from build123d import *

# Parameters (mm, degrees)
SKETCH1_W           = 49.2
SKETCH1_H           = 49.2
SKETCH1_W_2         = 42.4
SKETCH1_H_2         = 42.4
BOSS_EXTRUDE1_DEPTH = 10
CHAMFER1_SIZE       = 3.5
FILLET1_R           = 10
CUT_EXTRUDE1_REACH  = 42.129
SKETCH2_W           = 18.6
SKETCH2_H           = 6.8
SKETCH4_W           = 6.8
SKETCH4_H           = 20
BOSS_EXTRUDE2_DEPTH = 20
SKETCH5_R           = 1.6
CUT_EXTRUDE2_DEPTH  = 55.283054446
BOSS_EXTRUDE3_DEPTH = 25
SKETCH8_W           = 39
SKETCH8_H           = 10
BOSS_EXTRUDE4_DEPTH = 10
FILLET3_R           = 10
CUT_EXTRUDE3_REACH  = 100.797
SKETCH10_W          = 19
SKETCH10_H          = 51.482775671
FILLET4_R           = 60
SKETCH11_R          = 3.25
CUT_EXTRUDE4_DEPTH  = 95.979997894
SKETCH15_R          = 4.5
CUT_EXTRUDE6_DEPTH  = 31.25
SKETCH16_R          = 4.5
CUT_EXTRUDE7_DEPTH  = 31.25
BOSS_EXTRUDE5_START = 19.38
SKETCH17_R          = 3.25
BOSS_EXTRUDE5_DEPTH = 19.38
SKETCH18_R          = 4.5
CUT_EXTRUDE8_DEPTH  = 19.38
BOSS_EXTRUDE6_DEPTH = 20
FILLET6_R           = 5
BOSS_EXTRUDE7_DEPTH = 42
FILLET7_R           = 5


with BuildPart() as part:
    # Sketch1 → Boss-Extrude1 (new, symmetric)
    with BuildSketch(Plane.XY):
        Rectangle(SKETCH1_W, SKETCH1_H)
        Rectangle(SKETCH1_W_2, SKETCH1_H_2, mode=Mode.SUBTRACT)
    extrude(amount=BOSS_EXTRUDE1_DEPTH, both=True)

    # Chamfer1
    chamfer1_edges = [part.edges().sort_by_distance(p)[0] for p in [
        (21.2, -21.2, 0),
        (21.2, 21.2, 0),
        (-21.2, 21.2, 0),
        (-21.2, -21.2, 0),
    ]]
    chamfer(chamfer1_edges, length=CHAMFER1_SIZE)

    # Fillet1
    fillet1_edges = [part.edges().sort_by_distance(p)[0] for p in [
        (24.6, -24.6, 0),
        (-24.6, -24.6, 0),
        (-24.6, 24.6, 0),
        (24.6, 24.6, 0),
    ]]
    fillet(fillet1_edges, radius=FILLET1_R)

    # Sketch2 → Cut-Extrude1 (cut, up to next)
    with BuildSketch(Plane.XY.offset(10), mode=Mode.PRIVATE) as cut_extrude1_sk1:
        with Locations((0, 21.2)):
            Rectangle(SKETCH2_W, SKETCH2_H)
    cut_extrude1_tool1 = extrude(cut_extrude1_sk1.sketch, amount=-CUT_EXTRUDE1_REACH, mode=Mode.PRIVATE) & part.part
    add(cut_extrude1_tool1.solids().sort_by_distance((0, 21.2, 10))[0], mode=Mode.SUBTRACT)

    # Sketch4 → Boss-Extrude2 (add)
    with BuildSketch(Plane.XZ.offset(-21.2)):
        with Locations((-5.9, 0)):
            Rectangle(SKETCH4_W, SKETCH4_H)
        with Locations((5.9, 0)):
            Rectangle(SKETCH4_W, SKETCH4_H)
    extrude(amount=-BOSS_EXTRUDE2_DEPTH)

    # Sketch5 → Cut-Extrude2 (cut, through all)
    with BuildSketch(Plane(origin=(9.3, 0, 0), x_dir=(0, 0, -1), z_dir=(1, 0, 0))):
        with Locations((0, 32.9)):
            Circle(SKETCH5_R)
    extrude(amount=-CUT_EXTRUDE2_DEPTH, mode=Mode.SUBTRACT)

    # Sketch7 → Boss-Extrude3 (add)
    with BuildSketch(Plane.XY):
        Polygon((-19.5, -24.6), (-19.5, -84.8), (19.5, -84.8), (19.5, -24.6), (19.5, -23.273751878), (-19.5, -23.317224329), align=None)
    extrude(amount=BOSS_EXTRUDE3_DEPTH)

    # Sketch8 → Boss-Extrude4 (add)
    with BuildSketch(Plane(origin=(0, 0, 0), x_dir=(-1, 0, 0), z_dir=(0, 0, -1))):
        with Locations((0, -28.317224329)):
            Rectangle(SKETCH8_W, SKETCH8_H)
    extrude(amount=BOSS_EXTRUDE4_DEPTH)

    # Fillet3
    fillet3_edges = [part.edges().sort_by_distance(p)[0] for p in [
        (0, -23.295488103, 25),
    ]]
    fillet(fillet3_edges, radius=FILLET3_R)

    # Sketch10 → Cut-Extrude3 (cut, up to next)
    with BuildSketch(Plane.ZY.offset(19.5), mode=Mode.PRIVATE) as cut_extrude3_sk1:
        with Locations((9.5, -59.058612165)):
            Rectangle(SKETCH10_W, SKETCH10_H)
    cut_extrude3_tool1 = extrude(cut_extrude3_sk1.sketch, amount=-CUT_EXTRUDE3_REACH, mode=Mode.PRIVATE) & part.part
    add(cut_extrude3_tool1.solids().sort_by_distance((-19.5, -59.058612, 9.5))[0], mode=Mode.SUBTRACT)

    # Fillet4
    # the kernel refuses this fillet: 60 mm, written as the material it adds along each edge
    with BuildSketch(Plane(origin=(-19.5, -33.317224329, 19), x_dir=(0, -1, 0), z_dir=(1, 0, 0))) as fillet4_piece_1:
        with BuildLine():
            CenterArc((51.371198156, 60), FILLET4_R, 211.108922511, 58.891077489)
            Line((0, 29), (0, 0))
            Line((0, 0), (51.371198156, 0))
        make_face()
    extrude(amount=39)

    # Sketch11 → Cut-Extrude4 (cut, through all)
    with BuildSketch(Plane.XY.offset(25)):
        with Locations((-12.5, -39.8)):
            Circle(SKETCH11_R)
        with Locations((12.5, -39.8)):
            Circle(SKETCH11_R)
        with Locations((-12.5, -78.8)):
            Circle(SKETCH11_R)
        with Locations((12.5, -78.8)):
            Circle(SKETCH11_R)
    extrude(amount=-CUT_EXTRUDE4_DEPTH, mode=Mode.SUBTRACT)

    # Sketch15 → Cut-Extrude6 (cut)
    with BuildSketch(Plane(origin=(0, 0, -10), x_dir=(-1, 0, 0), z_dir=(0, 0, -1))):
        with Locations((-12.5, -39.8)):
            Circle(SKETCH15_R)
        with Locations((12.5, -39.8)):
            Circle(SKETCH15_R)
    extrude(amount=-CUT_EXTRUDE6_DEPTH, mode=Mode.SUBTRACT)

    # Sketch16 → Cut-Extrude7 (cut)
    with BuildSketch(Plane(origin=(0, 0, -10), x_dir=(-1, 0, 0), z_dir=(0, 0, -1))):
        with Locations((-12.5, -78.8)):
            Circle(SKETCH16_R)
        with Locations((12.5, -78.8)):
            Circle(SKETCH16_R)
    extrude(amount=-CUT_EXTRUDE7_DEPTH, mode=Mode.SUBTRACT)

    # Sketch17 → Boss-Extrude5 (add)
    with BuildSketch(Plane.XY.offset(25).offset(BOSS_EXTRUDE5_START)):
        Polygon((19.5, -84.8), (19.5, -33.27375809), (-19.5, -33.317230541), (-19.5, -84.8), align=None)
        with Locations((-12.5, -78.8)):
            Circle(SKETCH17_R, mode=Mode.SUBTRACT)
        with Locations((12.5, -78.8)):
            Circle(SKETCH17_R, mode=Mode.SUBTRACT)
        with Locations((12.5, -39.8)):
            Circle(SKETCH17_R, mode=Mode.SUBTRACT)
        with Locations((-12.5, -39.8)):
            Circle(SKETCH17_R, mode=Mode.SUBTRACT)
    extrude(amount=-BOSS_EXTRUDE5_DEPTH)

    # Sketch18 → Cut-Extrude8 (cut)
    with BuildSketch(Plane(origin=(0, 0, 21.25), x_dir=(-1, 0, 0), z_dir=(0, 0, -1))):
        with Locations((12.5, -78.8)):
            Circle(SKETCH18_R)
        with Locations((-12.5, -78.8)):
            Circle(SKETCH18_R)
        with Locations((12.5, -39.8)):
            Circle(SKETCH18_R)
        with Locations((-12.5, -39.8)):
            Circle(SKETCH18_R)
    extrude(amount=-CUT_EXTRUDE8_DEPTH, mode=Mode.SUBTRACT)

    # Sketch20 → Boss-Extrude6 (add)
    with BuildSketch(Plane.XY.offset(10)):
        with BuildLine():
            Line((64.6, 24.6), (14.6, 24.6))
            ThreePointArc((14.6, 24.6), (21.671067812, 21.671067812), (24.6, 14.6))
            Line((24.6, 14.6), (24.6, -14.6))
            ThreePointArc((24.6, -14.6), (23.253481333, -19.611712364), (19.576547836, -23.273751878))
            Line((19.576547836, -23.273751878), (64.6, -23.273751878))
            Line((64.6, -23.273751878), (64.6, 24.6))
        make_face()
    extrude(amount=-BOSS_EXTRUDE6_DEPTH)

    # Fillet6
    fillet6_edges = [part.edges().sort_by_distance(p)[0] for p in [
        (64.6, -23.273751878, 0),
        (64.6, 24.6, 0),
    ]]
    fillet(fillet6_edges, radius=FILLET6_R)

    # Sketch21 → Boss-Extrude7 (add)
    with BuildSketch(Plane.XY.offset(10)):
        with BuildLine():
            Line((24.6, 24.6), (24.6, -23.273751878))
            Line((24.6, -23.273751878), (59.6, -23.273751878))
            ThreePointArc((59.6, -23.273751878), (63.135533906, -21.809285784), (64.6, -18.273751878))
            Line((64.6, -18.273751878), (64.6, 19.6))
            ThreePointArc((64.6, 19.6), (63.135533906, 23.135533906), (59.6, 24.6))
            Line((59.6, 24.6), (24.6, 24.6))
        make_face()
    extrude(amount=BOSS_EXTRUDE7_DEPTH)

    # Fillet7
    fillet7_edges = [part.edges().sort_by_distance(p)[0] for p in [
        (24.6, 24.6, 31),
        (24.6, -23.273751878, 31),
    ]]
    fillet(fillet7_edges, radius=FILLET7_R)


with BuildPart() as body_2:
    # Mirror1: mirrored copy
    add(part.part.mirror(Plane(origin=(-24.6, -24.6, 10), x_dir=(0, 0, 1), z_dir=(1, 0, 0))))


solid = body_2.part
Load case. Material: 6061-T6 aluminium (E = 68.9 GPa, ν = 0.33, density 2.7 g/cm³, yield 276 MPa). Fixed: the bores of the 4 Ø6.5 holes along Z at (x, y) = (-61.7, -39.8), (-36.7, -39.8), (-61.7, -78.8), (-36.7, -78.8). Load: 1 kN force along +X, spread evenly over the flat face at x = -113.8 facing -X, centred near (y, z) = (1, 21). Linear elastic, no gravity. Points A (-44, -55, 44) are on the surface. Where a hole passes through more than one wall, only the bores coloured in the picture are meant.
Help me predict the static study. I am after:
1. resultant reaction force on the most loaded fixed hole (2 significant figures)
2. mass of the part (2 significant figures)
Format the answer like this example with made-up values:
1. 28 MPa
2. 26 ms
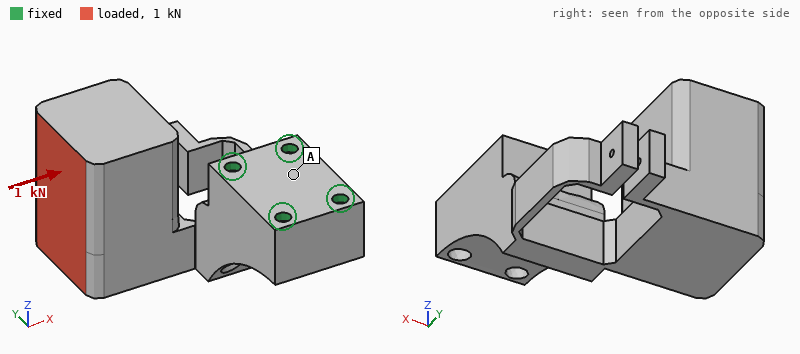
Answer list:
1. 950 N
2. 550 g
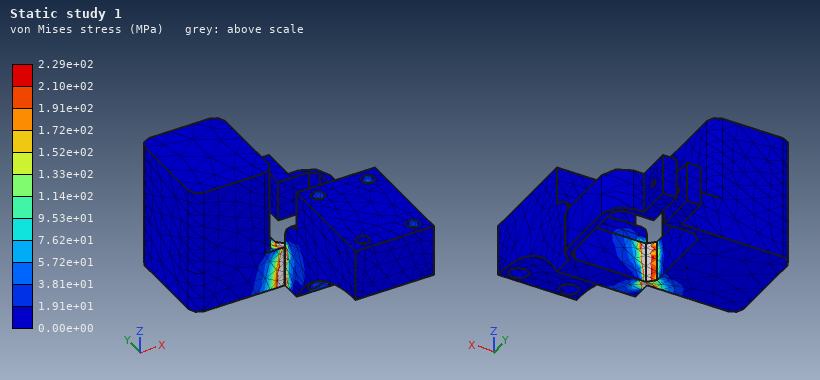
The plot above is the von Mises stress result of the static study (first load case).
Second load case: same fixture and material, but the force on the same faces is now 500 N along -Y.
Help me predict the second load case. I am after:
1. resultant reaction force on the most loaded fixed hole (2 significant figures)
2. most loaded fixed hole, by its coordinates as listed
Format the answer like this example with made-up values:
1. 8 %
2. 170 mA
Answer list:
1. 460 N
2. (-61.7, -39.8)
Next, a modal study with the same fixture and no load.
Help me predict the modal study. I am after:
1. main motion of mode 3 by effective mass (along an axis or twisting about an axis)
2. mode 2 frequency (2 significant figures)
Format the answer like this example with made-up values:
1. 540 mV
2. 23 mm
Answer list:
1. along Z
2. 400 Hz
